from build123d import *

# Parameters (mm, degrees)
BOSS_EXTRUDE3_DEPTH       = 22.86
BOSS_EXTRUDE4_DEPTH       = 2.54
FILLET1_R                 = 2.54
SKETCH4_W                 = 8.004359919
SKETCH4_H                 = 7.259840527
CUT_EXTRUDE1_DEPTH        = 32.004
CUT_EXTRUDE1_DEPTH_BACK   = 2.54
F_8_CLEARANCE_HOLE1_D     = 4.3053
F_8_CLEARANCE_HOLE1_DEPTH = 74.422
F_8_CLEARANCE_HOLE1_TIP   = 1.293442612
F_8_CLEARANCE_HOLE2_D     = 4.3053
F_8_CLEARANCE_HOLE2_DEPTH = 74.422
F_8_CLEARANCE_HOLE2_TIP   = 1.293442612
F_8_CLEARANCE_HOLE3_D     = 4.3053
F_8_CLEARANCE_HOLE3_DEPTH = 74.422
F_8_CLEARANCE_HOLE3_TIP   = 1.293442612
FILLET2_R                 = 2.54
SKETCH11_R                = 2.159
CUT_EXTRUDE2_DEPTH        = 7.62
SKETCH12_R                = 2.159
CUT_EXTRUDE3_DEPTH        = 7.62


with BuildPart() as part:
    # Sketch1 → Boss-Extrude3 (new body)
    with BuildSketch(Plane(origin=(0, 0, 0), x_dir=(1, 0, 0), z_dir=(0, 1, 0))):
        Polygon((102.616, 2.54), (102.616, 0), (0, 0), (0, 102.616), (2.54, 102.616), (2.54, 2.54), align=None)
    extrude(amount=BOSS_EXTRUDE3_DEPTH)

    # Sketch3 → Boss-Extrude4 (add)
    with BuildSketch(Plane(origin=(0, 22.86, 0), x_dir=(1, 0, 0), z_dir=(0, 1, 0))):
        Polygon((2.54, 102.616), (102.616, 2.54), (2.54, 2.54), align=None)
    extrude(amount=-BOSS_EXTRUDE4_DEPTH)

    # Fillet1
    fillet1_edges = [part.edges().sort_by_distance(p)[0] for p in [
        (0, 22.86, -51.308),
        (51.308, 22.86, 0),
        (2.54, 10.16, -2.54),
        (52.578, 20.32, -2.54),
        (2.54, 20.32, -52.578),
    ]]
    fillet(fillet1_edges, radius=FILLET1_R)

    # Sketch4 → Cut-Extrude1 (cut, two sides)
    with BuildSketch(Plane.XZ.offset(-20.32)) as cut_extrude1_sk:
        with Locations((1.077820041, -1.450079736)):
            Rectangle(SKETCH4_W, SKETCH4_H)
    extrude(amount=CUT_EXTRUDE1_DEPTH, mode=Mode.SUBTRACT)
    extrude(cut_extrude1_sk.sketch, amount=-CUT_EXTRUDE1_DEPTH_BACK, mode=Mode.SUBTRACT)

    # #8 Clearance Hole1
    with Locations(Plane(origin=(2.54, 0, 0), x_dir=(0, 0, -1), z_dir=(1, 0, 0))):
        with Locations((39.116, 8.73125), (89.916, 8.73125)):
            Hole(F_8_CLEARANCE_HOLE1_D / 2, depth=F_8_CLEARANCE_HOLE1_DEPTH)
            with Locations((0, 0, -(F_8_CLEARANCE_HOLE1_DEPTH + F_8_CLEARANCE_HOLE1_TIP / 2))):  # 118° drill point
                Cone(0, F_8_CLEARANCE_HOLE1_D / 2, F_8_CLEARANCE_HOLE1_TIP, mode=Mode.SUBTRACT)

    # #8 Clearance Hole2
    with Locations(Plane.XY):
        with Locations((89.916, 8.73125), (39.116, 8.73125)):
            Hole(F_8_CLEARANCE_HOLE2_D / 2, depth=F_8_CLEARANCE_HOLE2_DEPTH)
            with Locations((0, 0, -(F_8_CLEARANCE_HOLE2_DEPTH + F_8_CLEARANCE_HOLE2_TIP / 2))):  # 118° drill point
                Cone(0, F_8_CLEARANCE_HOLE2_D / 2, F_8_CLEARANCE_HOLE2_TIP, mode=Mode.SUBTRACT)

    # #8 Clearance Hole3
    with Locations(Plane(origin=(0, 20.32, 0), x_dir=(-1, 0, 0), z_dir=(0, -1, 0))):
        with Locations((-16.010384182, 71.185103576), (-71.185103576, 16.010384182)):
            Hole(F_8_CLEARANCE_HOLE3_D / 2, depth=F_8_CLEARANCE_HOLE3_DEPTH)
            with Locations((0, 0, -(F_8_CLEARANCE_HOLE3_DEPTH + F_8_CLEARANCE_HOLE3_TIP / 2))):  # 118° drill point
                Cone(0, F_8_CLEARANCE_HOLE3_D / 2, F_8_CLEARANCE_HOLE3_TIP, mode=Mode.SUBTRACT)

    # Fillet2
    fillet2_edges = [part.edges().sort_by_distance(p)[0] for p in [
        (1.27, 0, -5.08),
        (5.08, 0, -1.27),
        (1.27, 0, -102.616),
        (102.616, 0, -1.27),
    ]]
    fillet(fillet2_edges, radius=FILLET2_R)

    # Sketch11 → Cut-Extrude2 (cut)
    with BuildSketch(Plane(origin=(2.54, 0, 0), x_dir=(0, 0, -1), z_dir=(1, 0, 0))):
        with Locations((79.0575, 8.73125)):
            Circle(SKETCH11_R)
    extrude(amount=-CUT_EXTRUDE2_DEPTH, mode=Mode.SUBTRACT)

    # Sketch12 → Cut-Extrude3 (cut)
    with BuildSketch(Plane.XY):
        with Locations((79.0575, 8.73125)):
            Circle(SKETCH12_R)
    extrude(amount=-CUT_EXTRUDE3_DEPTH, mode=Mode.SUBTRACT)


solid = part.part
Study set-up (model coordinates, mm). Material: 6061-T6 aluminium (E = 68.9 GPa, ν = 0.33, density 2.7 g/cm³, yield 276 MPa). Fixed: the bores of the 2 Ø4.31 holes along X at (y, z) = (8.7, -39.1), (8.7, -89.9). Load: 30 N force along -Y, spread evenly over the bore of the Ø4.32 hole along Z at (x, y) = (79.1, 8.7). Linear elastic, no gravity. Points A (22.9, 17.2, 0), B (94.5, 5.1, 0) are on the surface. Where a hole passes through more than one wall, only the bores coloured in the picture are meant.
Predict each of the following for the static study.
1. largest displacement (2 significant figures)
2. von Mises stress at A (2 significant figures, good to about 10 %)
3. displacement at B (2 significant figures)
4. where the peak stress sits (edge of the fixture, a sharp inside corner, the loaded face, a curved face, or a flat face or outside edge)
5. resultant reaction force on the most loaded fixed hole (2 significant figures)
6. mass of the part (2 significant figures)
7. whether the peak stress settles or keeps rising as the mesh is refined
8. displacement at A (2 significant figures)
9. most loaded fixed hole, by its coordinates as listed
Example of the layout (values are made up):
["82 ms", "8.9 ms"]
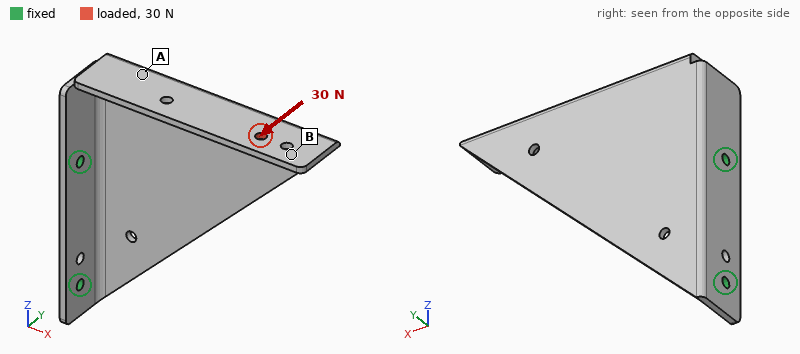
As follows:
["1.5 mm", "9.5 MPa", "1.4 mm", "edge of the fixture", "52 N", "64 g", "keeps rising", "0.31 mm", "(8.7, -39.1)"]
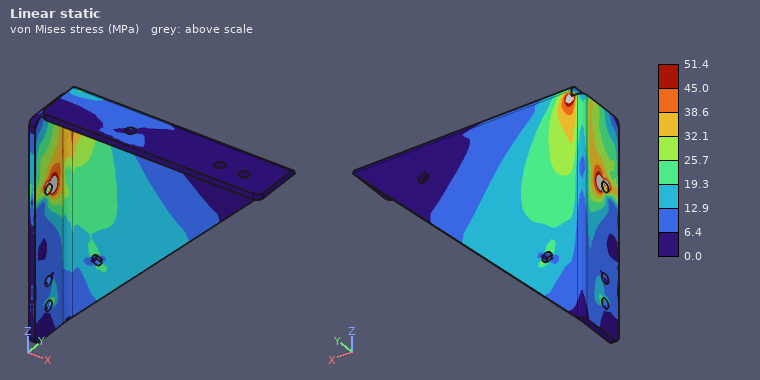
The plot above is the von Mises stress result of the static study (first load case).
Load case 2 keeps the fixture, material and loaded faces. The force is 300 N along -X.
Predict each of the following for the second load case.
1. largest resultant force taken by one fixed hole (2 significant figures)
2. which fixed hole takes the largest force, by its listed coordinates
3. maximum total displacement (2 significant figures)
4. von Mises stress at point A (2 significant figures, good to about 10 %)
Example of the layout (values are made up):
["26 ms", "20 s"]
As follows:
["490 N", "(8.7, -39.1)", "1.6 mm", "14 MPa"]
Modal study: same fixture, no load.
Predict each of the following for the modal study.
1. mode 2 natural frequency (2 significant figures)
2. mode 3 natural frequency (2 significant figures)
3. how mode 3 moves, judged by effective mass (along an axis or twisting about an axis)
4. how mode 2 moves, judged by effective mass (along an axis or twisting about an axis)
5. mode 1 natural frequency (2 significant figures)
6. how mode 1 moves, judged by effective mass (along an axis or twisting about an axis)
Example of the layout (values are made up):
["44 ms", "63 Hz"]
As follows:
["890 Hz", "970 Hz", "along X", "along Z", "210 Hz", "along Y"]
